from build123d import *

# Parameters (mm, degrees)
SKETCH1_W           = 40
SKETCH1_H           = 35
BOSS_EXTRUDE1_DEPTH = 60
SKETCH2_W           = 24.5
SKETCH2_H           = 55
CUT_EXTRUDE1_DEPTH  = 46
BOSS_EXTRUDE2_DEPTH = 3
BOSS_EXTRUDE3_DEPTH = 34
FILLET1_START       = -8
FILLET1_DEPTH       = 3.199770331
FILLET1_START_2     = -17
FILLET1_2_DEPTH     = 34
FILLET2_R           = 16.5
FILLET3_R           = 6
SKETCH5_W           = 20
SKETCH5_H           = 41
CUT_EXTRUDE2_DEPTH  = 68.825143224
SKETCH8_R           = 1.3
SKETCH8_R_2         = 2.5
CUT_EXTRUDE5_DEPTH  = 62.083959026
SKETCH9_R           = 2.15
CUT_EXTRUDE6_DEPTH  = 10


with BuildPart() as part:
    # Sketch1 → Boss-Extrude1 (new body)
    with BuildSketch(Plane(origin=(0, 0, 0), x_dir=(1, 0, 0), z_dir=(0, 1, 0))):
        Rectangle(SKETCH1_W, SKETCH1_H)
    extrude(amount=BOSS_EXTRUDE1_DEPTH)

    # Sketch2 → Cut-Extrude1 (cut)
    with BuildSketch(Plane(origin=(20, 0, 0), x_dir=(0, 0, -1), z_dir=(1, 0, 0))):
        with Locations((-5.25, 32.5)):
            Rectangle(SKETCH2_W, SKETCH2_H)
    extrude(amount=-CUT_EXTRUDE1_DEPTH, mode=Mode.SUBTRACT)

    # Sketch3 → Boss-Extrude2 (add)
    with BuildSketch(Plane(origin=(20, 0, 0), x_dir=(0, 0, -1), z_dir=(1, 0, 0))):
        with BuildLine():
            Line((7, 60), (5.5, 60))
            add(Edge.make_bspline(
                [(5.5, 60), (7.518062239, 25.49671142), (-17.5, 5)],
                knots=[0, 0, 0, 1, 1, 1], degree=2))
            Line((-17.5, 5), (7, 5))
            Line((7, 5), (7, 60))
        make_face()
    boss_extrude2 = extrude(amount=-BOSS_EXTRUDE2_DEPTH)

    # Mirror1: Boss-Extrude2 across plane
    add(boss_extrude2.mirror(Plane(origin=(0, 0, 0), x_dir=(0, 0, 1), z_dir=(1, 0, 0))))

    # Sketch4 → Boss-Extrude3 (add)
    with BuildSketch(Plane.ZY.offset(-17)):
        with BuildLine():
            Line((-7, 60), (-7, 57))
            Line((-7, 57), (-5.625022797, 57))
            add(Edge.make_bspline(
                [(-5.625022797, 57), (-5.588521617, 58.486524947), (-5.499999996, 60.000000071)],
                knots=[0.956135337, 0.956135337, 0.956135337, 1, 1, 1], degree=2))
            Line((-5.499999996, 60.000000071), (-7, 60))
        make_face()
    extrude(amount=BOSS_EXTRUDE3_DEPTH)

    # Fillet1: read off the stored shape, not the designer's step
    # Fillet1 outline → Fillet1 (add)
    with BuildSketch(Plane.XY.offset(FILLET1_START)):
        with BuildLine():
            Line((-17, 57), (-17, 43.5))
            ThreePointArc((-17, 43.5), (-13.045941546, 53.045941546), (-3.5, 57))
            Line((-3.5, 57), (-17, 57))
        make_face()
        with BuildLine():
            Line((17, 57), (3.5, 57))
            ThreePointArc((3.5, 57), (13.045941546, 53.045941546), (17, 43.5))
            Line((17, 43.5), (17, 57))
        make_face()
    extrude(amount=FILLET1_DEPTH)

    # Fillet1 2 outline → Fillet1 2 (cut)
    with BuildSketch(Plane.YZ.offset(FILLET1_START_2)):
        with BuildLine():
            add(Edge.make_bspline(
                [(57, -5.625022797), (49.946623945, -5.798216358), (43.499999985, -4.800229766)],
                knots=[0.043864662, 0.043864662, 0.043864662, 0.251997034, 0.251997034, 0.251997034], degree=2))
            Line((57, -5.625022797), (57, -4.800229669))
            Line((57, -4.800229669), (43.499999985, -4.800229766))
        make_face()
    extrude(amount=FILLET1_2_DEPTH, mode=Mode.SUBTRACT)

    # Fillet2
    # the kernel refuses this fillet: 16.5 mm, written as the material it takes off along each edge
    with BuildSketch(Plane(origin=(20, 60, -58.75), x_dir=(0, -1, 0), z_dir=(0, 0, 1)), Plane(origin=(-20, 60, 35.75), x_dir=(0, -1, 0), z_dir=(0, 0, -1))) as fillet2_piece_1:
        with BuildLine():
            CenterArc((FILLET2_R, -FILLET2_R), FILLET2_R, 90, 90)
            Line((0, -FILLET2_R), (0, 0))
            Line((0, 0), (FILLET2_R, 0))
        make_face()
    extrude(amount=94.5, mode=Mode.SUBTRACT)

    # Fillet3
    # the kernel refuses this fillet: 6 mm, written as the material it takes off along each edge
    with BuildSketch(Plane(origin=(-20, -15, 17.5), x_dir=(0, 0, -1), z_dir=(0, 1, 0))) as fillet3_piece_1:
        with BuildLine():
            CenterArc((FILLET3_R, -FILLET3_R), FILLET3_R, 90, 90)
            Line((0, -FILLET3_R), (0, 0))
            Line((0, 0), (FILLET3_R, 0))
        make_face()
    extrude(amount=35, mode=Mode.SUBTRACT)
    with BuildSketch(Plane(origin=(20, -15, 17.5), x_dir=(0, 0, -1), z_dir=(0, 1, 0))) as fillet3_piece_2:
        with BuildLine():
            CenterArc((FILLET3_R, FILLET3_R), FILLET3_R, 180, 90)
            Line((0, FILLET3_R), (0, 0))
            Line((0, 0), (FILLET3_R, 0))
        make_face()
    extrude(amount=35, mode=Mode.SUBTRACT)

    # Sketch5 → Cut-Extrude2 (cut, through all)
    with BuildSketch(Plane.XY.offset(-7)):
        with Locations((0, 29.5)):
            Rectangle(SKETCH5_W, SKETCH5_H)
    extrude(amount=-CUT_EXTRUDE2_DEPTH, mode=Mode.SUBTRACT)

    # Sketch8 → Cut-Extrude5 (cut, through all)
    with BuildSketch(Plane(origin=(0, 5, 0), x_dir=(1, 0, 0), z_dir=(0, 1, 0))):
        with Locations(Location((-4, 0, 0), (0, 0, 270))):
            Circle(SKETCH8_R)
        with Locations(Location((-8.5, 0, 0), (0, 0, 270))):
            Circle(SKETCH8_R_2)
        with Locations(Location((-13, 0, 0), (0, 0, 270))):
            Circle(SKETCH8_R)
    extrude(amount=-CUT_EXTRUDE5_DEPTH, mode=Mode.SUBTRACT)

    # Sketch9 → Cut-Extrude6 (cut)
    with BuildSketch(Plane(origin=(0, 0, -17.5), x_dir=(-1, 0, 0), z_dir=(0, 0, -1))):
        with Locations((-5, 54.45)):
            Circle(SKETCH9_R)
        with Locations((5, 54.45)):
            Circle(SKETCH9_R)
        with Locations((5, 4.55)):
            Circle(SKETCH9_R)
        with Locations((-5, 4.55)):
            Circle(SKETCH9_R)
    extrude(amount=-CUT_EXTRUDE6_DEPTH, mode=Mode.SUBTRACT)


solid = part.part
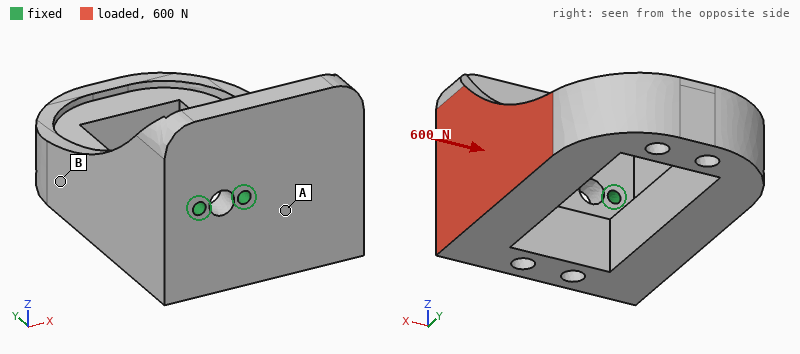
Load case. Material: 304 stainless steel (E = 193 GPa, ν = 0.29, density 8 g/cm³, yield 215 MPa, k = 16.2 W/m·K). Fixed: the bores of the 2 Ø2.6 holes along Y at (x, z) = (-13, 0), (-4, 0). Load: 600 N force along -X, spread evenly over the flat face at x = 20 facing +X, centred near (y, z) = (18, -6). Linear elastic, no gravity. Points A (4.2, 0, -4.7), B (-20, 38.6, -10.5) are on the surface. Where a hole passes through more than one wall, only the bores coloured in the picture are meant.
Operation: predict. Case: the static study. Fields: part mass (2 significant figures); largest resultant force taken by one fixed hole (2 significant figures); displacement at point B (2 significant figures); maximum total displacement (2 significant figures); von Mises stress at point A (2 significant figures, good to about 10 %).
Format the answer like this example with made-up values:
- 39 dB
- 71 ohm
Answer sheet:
- 180 g
- 750 N
- 23 µm
- 37 µm
- 13 MPa
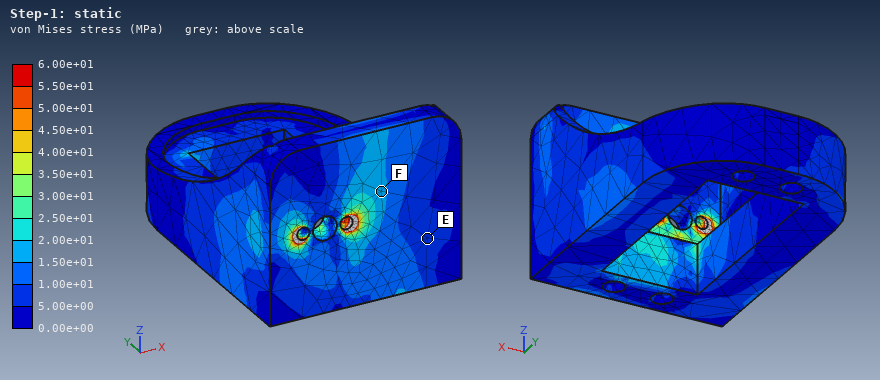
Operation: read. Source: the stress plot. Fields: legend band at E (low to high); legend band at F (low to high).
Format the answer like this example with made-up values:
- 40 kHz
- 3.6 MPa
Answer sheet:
- 5.00e+00 to 1.00e+01 MPa
- 1.50e+01 to 2.00e+01 MPa
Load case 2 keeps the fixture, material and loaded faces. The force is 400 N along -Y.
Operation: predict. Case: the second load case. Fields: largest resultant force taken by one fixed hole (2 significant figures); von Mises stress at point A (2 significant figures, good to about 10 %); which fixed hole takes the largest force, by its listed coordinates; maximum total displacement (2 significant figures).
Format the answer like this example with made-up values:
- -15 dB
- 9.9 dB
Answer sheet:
- 890 N
- 16 MPa
- (-4, 0)
- 36 µm
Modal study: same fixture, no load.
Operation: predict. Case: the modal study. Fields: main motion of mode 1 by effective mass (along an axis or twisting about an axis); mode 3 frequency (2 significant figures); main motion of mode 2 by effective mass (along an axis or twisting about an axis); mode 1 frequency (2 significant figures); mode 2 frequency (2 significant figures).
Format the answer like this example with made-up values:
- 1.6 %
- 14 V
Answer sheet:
- along Z
- 4100 Hz
- along X
- 1400 Hz
- 1600 Hz
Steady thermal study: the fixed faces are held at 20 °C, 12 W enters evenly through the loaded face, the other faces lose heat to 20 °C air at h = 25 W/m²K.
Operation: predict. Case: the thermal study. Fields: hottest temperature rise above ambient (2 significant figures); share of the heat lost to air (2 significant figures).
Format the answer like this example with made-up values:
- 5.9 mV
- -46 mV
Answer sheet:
- 76 K
- 56 %
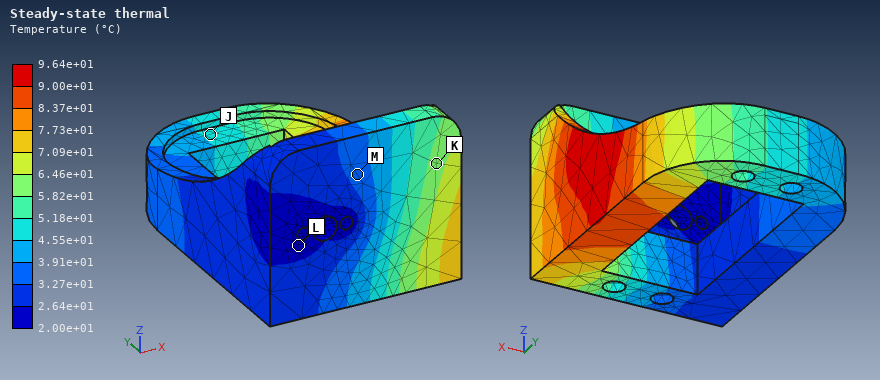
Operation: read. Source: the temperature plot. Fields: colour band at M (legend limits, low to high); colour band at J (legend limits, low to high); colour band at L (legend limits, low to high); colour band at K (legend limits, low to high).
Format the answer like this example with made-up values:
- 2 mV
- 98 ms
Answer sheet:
- 3.27e+01 to 3.91e+01 °C
- 4.55e+01 to 5.18e+01 °C
- 2.00e+01 to 2.64e+01 °C
- 5.82e+01 to 6.46e+01 °C
